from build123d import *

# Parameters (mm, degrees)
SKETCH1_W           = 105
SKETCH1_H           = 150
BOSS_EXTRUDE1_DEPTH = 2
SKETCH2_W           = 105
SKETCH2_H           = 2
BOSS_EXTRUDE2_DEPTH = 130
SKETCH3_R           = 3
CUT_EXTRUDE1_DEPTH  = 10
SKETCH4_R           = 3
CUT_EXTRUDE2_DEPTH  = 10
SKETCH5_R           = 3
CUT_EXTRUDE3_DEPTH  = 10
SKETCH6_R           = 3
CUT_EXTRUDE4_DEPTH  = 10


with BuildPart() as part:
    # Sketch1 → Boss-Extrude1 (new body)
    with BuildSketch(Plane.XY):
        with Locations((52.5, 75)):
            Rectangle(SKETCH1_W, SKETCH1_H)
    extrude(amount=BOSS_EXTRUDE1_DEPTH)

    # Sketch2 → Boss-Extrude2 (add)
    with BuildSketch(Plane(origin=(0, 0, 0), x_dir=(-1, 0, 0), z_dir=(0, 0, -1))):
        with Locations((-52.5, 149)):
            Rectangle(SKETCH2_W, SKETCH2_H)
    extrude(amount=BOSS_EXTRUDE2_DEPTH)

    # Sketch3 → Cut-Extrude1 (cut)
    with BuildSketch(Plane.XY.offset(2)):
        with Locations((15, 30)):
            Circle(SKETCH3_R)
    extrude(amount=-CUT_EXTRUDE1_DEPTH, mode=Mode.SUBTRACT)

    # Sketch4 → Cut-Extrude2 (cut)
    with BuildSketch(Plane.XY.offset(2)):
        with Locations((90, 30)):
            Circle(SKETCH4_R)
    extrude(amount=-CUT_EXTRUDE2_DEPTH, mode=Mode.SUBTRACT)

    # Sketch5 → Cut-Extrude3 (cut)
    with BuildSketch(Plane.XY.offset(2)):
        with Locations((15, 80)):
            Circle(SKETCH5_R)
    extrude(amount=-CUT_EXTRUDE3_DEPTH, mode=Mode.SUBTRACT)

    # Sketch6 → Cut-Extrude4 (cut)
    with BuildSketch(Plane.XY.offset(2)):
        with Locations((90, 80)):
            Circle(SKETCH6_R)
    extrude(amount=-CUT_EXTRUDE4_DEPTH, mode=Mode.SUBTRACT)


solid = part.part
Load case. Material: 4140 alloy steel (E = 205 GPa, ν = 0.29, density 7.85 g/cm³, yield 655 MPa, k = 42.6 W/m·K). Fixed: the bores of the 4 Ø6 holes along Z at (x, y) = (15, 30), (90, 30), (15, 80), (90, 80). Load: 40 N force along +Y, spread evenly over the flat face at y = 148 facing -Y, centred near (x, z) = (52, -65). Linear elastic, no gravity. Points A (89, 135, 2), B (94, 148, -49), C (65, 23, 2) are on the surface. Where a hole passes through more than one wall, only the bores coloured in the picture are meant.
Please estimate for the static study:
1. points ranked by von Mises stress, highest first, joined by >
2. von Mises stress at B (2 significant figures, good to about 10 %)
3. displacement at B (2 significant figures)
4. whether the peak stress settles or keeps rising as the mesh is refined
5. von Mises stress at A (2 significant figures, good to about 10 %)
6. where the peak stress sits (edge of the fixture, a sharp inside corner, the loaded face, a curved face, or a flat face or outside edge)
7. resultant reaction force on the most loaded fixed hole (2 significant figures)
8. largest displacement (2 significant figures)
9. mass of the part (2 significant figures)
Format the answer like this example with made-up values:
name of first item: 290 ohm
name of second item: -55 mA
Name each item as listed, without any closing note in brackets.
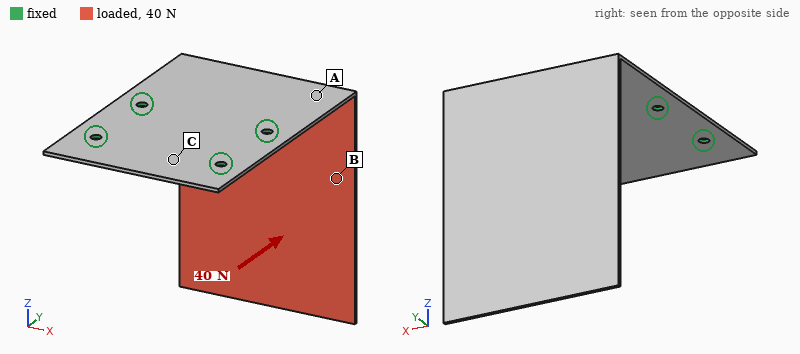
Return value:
points ranked by von Mises stress, highest first, joined by >: A > B > C
von Mises stress at B: 14 MPa
displacement at B: 0.88 mm
whether the peak stress settles or keeps rising as the mesh is refined: keeps rising
von Mises stress at A: 34 MPa
where the peak stress sits: edge of the fixture
resultant reaction force on the most loaded fixed hole: 17 N
largest displacement: 2.4 mm
mass of the part: 460 g
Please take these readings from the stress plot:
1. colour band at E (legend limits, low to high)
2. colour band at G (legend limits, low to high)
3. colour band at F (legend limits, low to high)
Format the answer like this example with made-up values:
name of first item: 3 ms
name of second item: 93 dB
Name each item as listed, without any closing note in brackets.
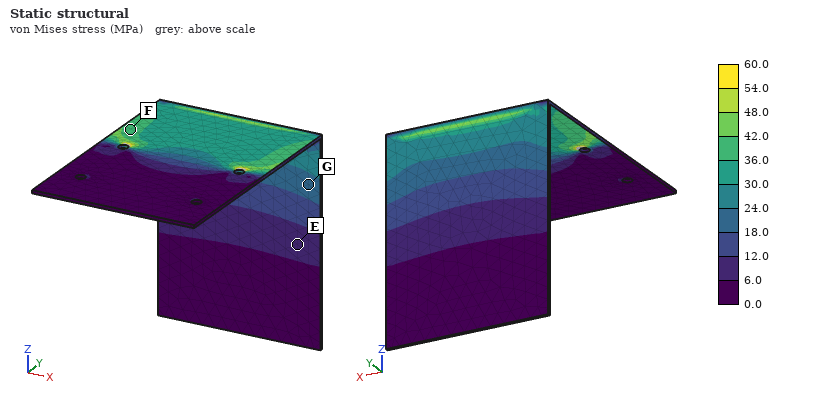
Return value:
colour band at E: 6.0 to 12.0 MPa
colour band at G: 18.0 to 24.0 MPa
colour band at F: 36.0 to 42.0 MPa
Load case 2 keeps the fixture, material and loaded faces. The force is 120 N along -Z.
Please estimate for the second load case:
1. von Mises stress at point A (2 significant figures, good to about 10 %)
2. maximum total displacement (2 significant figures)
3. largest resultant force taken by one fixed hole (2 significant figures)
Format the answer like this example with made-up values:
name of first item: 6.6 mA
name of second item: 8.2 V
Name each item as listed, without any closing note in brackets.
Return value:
von Mises stress at point A: 24 MPa
maximum total displacement: 2.7 mm
largest resultant force taken by one fixed hole: 82 N
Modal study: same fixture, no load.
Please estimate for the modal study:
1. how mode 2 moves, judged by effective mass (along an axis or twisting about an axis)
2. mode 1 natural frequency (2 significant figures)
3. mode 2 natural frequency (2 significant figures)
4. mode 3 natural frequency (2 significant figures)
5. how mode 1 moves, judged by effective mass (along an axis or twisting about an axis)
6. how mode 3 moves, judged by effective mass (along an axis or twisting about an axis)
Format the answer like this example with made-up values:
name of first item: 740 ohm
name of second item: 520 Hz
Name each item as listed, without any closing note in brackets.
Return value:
how mode 2 moves, judged by effective mass: along X
mode 1 natural frequency: 52 Hz
mode 2 natural frequency: 110 Hz
mode 3 natural frequency: 170 Hz
how mode 1 moves, judged by effective mass: along Y
how mode 3 moves, judged by effective mass: along Z
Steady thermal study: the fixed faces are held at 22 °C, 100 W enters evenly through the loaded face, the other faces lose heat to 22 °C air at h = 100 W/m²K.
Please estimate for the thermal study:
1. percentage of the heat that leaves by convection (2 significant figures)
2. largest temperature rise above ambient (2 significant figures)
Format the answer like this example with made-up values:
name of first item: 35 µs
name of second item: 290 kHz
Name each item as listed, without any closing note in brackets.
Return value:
percentage of the heat that leaves by convection: 100 %
largest temperature rise above ambient: 69 K
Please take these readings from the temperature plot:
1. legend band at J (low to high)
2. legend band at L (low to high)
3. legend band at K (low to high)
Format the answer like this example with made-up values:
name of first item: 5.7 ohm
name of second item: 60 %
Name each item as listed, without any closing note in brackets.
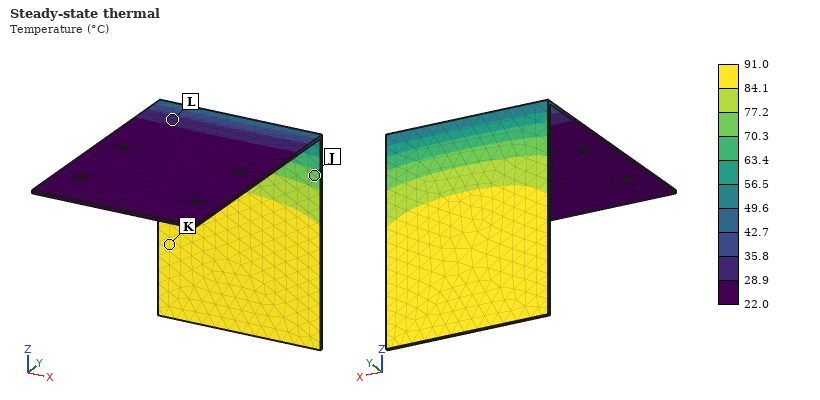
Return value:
legend band at J: 70.3 to 77.2 °C
legend band at L: 28.9 to 35.8 °C
legend band at K: 84.1 to 91.0 °C
